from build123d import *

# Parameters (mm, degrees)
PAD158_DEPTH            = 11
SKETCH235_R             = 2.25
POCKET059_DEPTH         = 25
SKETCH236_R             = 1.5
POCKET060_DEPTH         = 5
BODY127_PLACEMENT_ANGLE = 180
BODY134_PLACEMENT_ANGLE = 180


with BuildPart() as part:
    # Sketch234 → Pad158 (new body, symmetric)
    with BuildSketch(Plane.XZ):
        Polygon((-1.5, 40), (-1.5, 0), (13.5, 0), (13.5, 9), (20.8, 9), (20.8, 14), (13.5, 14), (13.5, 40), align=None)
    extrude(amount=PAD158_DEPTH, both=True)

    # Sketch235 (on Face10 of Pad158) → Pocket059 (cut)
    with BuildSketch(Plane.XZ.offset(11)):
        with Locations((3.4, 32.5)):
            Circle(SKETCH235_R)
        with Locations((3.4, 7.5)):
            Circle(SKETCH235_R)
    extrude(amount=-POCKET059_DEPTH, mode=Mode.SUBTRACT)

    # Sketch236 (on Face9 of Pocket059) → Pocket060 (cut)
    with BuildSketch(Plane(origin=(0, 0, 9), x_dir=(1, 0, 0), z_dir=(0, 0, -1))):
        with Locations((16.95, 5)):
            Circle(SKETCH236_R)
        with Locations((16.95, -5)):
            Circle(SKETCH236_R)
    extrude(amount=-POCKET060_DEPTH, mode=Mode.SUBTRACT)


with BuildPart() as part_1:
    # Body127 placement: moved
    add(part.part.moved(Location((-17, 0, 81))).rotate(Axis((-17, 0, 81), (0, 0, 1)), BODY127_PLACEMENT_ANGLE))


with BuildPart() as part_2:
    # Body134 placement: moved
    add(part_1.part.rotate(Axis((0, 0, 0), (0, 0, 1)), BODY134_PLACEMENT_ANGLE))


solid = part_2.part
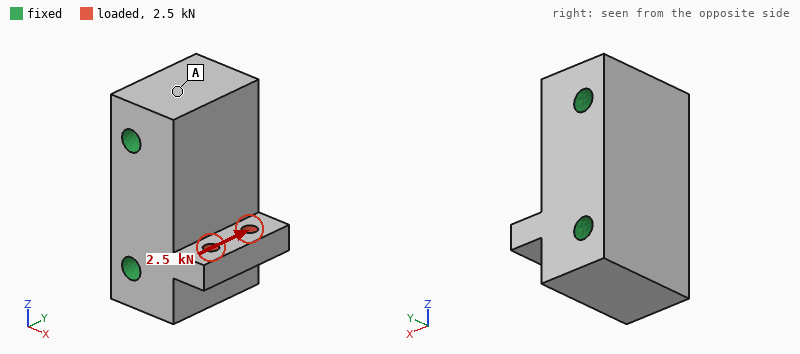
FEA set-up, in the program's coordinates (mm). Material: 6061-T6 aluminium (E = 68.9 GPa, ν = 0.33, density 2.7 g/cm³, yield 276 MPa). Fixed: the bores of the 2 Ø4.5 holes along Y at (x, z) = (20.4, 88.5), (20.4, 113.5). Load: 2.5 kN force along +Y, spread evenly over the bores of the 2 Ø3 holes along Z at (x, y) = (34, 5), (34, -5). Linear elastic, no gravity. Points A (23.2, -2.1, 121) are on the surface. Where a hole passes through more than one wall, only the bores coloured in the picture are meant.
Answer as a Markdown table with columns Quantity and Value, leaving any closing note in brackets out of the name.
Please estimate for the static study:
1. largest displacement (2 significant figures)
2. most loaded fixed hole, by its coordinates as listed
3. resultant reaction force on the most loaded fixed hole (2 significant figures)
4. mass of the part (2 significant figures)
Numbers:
| Quantity | Value |
|---|---|
| largest displacement | 16 µm |
| most loaded fixed hole, by its coordinates as listed | (20.4, 88.5) |
| resultant reaction force on the most loaded fixed hole | 2.1 kN |
| mass of the part | 36 g |
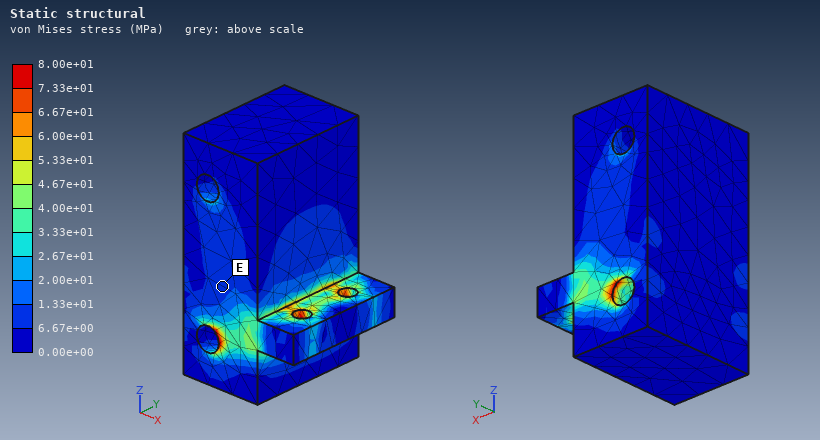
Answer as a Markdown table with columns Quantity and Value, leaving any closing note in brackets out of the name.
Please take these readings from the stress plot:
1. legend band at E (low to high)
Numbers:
| Quantity | Value |
|---|---|
| legend band at E | 6.67e+00 to 1.33e+01 MPa |
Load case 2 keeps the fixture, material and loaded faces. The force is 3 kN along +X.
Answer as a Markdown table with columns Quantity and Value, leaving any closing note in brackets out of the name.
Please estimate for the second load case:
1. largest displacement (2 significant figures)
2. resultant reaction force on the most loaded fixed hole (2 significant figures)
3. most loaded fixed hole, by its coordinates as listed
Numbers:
| Quantity | Value |
|---|---|
| largest displacement | 6.8 µm |
| resultant reaction force on the most loaded fixed hole | 2.6 kN |
| most loaded fixed hole, by its coordinates as listed | (20.4, 88.5) |
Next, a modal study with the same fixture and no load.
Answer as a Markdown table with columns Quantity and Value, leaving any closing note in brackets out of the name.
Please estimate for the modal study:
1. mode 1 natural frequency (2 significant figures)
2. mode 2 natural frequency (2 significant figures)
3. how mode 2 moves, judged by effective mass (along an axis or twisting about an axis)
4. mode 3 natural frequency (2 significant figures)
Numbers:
| Quantity | Value |
|---|---|
| mode 1 natural frequency | 37 kHz |
| mode 2 natural frequency | 41 kHz |
| how mode 2 moves, judged by effective mass | along Y |
| mode 3 natural frequency | 50 kHz |
